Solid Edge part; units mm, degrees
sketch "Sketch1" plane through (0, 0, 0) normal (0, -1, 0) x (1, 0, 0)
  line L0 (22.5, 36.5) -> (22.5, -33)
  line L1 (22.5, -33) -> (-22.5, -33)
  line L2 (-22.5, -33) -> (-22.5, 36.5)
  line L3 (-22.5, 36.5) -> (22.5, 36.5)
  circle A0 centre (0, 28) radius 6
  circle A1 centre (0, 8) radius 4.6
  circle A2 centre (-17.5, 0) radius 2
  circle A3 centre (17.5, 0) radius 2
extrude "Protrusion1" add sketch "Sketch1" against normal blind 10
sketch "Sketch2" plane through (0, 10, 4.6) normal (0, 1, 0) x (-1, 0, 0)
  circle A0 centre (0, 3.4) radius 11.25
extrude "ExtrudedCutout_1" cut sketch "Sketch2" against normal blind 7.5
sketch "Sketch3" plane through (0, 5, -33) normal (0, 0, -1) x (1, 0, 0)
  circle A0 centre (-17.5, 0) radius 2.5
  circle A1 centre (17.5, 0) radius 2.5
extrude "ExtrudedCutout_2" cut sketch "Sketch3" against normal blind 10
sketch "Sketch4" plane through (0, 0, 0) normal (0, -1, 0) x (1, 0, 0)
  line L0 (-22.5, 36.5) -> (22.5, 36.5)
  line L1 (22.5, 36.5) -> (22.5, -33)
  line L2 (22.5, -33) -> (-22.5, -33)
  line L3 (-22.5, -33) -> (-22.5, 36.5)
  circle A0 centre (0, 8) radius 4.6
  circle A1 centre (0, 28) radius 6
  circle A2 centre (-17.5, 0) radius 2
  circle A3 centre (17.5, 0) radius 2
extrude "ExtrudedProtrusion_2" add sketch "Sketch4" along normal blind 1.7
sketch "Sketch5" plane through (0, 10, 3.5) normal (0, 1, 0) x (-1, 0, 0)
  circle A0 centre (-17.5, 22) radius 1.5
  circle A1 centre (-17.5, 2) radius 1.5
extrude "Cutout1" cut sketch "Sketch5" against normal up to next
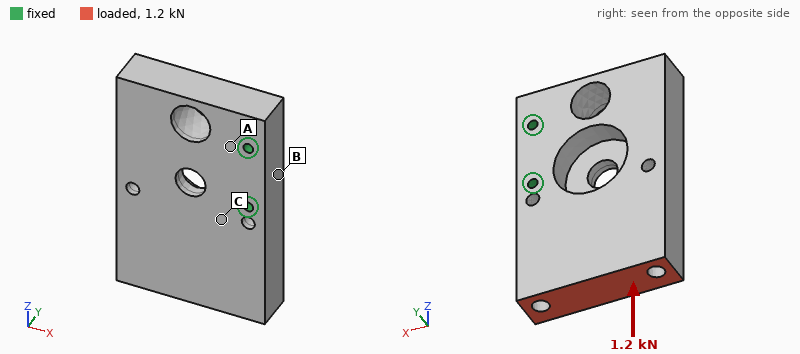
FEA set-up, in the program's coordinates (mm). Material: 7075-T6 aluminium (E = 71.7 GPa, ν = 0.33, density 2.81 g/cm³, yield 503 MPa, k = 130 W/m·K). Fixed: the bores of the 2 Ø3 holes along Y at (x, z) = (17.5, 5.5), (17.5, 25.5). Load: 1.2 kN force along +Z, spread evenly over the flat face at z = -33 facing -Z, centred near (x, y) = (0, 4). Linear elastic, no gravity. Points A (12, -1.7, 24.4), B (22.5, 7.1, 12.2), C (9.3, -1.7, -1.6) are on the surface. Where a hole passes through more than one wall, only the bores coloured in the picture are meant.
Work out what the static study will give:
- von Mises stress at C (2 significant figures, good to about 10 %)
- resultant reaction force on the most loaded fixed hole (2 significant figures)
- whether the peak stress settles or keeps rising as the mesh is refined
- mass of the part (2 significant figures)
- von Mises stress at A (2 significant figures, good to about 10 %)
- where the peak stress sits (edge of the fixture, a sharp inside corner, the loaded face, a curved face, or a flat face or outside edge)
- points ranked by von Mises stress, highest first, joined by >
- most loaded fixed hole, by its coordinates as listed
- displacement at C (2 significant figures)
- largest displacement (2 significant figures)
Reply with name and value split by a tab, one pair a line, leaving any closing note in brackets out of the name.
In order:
von Mises stress at C	5.9 MPa
resultant reaction force on the most loaded fixed hole	1.2 kN
whether the peak stress settles or keeps rising as the mesh is refined	keeps rising
mass of the part	88 g
von Mises stress at A	10 MPa
where the peak stress sits	edge of the fixture
points ranked by von Mises stress, highest first, joined by >	A > C > B
most loaded fixed hole, by its coordinates as listed	(17.5, 5.5)
displacement at C	4.6 µm
largest displacement	23 µm
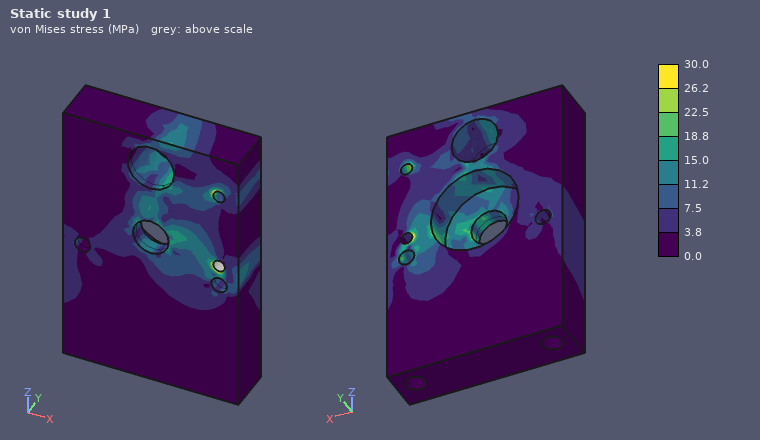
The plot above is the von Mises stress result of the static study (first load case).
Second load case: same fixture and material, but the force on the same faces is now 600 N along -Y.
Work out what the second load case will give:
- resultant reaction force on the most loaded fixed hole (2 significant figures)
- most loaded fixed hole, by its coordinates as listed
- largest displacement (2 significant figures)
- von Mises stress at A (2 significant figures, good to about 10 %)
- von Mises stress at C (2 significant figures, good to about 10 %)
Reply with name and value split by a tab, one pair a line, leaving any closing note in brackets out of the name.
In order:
resultant reaction force on the most loaded fixed hole	1.0 kN
most loaded fixed hole, by its coordinates as listed	(17.5, 5.5)
largest displacement	0.12 mm
von Mises stress at A	13 MPa
von Mises stress at C	35 MPa
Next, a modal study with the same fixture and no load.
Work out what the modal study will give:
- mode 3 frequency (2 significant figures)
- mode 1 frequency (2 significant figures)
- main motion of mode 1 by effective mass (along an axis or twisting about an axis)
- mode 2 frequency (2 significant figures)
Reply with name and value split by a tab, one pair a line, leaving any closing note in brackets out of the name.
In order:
mode 3 frequency	4600 Hz
mode 1 frequency	2600 Hz
main motion of mode 1 by effective mass	along Y
mode 2 frequency	4000 Hz
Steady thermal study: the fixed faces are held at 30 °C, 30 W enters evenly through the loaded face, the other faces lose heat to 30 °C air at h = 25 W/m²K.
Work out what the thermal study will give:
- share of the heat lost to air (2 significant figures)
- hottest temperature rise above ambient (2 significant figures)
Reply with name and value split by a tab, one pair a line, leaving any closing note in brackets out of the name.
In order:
share of the heat lost to air	10 %
hottest temperature rise above ambient	28 K
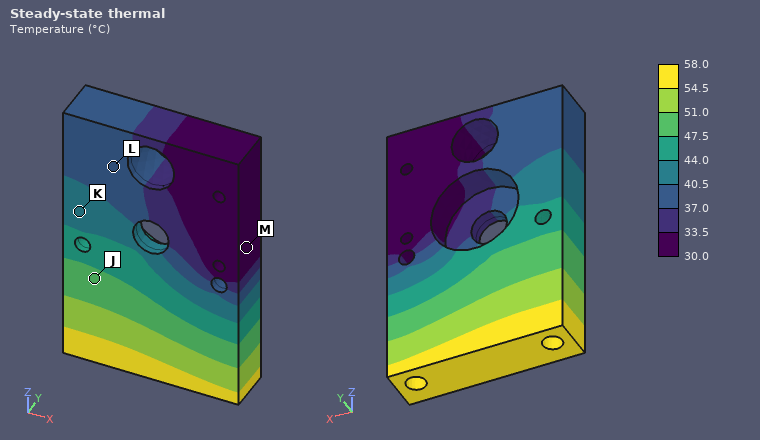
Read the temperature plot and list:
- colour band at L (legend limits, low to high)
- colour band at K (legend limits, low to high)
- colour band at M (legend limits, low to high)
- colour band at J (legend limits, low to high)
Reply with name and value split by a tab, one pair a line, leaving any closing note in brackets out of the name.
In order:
colour band at L	37.0 to 40.5 °C
colour band at K	40.5 to 44.0 °C
colour band at M	30.0 to 33.5 °C
colour band at J	47.5 to 51.0 °C
